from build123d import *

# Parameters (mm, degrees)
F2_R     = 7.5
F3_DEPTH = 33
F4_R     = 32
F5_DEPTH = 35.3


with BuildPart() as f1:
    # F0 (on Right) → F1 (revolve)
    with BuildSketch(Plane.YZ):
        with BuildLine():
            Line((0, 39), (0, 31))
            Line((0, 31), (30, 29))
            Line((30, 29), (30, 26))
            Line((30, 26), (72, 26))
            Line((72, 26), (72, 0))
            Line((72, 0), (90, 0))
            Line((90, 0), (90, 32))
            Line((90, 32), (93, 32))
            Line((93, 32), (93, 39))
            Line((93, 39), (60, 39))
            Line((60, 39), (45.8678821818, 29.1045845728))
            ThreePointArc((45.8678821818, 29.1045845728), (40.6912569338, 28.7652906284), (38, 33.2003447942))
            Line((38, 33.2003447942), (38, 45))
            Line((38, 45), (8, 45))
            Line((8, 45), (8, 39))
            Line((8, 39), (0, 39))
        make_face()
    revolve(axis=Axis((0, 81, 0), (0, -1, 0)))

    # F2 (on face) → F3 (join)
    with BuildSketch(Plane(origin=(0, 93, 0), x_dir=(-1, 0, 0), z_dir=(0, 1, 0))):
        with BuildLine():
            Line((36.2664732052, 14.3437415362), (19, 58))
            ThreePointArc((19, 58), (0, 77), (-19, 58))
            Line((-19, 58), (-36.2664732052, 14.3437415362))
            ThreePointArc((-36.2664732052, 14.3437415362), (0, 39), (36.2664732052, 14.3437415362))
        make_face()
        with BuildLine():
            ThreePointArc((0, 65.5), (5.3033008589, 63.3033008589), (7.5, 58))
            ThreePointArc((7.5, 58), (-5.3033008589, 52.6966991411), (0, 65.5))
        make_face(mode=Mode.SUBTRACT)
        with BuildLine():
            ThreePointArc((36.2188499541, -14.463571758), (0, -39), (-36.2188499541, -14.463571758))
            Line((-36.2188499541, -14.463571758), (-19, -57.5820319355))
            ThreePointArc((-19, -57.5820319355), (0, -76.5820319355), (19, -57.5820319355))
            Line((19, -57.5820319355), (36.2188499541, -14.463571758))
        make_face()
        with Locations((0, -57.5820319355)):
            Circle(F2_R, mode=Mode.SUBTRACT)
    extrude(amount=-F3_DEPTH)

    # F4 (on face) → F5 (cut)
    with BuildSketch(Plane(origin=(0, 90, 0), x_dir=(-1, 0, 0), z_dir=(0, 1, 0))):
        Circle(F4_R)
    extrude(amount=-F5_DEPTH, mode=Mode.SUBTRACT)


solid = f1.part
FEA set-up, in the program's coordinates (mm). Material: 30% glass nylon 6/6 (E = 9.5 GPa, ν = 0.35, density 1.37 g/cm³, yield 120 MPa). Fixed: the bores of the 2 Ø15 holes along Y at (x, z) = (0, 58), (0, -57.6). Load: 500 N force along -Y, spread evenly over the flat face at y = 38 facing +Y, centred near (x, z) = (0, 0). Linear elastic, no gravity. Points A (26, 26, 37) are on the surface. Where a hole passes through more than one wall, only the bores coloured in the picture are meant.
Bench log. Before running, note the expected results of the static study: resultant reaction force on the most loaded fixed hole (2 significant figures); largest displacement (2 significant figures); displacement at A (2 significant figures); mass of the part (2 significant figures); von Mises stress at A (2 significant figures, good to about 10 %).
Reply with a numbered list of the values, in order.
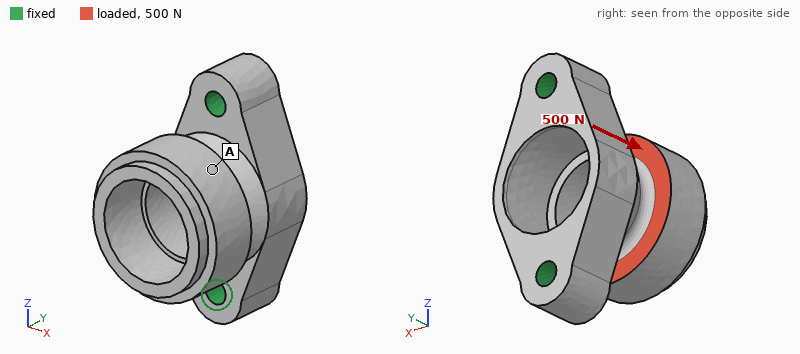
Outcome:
1. 260 N
2. 12 µm
3. 10 µm
4. 410 g
5. 0.32 MPa
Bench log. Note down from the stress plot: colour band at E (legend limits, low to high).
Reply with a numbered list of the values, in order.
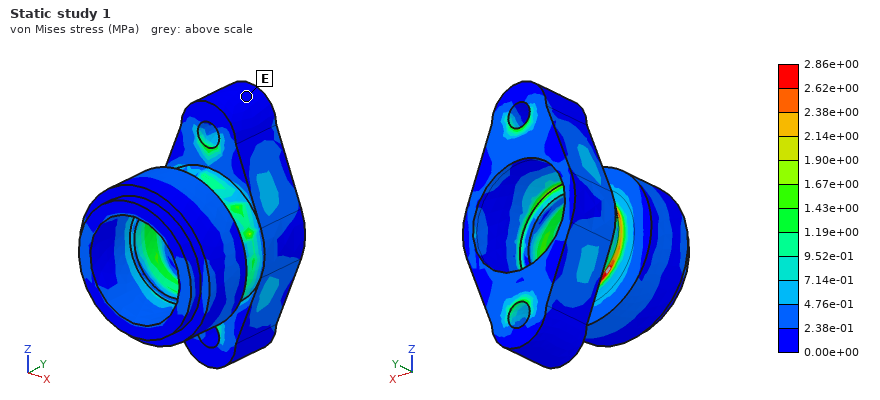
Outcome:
1. 0.00e+00 to 2.38e-01 MPa
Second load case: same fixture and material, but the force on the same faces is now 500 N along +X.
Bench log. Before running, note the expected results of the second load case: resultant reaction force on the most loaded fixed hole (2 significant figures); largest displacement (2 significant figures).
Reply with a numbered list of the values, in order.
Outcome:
1. 250 N
2. 35 µm
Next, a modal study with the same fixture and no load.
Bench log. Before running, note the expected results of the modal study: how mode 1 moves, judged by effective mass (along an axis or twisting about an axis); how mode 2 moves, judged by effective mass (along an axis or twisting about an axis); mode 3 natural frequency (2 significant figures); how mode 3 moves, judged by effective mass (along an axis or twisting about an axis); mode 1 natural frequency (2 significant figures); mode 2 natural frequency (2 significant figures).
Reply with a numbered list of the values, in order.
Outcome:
1. along X
2. along Z
3. 2500 Hz
4. twisting about Y
5. 1100 Hz
6. 1700 Hz
